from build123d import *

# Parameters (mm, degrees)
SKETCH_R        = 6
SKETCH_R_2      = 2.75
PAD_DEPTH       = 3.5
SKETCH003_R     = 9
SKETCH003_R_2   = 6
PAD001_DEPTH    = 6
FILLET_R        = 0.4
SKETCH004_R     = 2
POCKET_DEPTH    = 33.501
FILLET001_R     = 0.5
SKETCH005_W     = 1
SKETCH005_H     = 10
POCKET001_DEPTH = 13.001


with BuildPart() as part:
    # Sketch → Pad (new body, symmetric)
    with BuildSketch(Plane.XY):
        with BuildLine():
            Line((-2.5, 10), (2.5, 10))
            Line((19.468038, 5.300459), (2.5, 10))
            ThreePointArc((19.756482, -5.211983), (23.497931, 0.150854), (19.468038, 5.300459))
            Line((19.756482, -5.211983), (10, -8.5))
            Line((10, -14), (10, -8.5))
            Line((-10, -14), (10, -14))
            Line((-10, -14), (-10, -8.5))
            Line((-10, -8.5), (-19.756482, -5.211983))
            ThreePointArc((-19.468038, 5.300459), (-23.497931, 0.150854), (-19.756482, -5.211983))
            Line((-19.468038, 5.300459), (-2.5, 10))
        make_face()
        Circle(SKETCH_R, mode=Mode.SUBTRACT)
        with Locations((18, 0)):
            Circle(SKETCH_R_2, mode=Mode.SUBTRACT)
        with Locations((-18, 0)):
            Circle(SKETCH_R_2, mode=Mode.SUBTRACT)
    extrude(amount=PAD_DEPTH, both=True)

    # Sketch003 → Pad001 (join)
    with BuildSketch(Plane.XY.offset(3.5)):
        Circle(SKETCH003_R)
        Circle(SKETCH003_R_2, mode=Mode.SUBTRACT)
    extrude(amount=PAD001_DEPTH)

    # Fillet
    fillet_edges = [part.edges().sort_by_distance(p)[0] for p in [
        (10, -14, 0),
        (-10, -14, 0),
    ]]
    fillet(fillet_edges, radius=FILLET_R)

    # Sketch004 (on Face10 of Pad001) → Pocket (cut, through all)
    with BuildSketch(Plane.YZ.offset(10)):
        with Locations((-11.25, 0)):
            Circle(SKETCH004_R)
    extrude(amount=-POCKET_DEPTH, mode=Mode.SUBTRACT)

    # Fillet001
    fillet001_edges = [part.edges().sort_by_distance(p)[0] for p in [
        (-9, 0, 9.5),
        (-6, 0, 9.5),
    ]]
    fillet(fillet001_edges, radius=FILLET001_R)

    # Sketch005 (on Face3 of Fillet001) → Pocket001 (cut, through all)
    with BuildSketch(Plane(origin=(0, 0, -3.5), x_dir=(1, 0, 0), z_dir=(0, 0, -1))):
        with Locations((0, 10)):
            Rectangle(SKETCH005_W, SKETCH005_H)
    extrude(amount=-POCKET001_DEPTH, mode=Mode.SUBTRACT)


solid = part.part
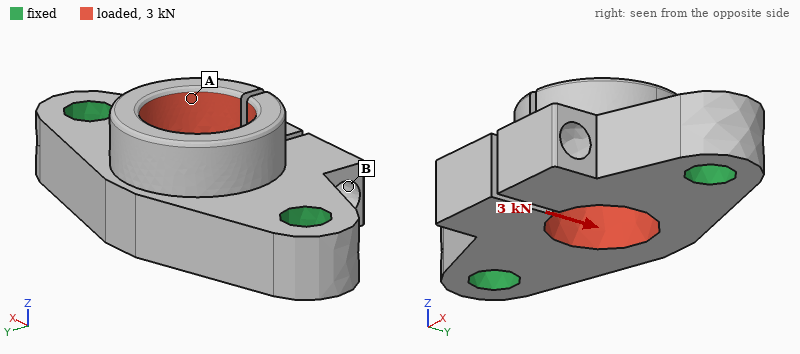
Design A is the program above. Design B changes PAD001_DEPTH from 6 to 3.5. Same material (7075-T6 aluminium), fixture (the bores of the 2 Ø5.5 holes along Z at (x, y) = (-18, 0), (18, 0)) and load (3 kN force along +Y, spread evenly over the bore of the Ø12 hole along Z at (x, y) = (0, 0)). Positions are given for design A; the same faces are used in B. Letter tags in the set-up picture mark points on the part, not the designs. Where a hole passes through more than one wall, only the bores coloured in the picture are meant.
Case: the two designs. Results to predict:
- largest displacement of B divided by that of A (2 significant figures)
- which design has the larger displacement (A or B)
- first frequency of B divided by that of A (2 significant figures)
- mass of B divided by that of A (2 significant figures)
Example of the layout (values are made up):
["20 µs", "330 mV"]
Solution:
["0.84", "A", "1.1", "0.93"]
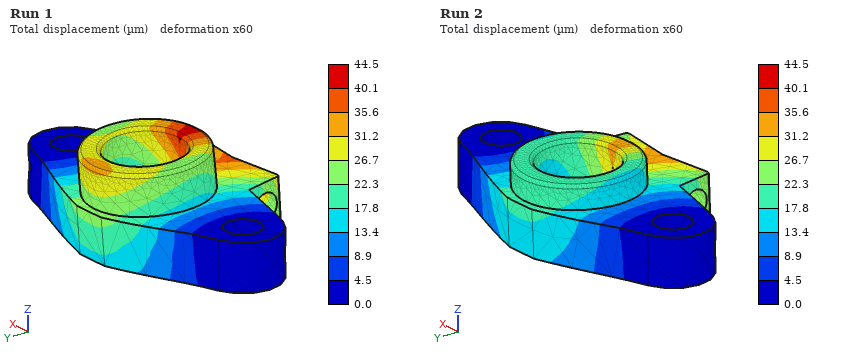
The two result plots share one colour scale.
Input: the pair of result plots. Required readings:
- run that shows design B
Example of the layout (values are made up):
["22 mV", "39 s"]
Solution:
["Run 2"]
